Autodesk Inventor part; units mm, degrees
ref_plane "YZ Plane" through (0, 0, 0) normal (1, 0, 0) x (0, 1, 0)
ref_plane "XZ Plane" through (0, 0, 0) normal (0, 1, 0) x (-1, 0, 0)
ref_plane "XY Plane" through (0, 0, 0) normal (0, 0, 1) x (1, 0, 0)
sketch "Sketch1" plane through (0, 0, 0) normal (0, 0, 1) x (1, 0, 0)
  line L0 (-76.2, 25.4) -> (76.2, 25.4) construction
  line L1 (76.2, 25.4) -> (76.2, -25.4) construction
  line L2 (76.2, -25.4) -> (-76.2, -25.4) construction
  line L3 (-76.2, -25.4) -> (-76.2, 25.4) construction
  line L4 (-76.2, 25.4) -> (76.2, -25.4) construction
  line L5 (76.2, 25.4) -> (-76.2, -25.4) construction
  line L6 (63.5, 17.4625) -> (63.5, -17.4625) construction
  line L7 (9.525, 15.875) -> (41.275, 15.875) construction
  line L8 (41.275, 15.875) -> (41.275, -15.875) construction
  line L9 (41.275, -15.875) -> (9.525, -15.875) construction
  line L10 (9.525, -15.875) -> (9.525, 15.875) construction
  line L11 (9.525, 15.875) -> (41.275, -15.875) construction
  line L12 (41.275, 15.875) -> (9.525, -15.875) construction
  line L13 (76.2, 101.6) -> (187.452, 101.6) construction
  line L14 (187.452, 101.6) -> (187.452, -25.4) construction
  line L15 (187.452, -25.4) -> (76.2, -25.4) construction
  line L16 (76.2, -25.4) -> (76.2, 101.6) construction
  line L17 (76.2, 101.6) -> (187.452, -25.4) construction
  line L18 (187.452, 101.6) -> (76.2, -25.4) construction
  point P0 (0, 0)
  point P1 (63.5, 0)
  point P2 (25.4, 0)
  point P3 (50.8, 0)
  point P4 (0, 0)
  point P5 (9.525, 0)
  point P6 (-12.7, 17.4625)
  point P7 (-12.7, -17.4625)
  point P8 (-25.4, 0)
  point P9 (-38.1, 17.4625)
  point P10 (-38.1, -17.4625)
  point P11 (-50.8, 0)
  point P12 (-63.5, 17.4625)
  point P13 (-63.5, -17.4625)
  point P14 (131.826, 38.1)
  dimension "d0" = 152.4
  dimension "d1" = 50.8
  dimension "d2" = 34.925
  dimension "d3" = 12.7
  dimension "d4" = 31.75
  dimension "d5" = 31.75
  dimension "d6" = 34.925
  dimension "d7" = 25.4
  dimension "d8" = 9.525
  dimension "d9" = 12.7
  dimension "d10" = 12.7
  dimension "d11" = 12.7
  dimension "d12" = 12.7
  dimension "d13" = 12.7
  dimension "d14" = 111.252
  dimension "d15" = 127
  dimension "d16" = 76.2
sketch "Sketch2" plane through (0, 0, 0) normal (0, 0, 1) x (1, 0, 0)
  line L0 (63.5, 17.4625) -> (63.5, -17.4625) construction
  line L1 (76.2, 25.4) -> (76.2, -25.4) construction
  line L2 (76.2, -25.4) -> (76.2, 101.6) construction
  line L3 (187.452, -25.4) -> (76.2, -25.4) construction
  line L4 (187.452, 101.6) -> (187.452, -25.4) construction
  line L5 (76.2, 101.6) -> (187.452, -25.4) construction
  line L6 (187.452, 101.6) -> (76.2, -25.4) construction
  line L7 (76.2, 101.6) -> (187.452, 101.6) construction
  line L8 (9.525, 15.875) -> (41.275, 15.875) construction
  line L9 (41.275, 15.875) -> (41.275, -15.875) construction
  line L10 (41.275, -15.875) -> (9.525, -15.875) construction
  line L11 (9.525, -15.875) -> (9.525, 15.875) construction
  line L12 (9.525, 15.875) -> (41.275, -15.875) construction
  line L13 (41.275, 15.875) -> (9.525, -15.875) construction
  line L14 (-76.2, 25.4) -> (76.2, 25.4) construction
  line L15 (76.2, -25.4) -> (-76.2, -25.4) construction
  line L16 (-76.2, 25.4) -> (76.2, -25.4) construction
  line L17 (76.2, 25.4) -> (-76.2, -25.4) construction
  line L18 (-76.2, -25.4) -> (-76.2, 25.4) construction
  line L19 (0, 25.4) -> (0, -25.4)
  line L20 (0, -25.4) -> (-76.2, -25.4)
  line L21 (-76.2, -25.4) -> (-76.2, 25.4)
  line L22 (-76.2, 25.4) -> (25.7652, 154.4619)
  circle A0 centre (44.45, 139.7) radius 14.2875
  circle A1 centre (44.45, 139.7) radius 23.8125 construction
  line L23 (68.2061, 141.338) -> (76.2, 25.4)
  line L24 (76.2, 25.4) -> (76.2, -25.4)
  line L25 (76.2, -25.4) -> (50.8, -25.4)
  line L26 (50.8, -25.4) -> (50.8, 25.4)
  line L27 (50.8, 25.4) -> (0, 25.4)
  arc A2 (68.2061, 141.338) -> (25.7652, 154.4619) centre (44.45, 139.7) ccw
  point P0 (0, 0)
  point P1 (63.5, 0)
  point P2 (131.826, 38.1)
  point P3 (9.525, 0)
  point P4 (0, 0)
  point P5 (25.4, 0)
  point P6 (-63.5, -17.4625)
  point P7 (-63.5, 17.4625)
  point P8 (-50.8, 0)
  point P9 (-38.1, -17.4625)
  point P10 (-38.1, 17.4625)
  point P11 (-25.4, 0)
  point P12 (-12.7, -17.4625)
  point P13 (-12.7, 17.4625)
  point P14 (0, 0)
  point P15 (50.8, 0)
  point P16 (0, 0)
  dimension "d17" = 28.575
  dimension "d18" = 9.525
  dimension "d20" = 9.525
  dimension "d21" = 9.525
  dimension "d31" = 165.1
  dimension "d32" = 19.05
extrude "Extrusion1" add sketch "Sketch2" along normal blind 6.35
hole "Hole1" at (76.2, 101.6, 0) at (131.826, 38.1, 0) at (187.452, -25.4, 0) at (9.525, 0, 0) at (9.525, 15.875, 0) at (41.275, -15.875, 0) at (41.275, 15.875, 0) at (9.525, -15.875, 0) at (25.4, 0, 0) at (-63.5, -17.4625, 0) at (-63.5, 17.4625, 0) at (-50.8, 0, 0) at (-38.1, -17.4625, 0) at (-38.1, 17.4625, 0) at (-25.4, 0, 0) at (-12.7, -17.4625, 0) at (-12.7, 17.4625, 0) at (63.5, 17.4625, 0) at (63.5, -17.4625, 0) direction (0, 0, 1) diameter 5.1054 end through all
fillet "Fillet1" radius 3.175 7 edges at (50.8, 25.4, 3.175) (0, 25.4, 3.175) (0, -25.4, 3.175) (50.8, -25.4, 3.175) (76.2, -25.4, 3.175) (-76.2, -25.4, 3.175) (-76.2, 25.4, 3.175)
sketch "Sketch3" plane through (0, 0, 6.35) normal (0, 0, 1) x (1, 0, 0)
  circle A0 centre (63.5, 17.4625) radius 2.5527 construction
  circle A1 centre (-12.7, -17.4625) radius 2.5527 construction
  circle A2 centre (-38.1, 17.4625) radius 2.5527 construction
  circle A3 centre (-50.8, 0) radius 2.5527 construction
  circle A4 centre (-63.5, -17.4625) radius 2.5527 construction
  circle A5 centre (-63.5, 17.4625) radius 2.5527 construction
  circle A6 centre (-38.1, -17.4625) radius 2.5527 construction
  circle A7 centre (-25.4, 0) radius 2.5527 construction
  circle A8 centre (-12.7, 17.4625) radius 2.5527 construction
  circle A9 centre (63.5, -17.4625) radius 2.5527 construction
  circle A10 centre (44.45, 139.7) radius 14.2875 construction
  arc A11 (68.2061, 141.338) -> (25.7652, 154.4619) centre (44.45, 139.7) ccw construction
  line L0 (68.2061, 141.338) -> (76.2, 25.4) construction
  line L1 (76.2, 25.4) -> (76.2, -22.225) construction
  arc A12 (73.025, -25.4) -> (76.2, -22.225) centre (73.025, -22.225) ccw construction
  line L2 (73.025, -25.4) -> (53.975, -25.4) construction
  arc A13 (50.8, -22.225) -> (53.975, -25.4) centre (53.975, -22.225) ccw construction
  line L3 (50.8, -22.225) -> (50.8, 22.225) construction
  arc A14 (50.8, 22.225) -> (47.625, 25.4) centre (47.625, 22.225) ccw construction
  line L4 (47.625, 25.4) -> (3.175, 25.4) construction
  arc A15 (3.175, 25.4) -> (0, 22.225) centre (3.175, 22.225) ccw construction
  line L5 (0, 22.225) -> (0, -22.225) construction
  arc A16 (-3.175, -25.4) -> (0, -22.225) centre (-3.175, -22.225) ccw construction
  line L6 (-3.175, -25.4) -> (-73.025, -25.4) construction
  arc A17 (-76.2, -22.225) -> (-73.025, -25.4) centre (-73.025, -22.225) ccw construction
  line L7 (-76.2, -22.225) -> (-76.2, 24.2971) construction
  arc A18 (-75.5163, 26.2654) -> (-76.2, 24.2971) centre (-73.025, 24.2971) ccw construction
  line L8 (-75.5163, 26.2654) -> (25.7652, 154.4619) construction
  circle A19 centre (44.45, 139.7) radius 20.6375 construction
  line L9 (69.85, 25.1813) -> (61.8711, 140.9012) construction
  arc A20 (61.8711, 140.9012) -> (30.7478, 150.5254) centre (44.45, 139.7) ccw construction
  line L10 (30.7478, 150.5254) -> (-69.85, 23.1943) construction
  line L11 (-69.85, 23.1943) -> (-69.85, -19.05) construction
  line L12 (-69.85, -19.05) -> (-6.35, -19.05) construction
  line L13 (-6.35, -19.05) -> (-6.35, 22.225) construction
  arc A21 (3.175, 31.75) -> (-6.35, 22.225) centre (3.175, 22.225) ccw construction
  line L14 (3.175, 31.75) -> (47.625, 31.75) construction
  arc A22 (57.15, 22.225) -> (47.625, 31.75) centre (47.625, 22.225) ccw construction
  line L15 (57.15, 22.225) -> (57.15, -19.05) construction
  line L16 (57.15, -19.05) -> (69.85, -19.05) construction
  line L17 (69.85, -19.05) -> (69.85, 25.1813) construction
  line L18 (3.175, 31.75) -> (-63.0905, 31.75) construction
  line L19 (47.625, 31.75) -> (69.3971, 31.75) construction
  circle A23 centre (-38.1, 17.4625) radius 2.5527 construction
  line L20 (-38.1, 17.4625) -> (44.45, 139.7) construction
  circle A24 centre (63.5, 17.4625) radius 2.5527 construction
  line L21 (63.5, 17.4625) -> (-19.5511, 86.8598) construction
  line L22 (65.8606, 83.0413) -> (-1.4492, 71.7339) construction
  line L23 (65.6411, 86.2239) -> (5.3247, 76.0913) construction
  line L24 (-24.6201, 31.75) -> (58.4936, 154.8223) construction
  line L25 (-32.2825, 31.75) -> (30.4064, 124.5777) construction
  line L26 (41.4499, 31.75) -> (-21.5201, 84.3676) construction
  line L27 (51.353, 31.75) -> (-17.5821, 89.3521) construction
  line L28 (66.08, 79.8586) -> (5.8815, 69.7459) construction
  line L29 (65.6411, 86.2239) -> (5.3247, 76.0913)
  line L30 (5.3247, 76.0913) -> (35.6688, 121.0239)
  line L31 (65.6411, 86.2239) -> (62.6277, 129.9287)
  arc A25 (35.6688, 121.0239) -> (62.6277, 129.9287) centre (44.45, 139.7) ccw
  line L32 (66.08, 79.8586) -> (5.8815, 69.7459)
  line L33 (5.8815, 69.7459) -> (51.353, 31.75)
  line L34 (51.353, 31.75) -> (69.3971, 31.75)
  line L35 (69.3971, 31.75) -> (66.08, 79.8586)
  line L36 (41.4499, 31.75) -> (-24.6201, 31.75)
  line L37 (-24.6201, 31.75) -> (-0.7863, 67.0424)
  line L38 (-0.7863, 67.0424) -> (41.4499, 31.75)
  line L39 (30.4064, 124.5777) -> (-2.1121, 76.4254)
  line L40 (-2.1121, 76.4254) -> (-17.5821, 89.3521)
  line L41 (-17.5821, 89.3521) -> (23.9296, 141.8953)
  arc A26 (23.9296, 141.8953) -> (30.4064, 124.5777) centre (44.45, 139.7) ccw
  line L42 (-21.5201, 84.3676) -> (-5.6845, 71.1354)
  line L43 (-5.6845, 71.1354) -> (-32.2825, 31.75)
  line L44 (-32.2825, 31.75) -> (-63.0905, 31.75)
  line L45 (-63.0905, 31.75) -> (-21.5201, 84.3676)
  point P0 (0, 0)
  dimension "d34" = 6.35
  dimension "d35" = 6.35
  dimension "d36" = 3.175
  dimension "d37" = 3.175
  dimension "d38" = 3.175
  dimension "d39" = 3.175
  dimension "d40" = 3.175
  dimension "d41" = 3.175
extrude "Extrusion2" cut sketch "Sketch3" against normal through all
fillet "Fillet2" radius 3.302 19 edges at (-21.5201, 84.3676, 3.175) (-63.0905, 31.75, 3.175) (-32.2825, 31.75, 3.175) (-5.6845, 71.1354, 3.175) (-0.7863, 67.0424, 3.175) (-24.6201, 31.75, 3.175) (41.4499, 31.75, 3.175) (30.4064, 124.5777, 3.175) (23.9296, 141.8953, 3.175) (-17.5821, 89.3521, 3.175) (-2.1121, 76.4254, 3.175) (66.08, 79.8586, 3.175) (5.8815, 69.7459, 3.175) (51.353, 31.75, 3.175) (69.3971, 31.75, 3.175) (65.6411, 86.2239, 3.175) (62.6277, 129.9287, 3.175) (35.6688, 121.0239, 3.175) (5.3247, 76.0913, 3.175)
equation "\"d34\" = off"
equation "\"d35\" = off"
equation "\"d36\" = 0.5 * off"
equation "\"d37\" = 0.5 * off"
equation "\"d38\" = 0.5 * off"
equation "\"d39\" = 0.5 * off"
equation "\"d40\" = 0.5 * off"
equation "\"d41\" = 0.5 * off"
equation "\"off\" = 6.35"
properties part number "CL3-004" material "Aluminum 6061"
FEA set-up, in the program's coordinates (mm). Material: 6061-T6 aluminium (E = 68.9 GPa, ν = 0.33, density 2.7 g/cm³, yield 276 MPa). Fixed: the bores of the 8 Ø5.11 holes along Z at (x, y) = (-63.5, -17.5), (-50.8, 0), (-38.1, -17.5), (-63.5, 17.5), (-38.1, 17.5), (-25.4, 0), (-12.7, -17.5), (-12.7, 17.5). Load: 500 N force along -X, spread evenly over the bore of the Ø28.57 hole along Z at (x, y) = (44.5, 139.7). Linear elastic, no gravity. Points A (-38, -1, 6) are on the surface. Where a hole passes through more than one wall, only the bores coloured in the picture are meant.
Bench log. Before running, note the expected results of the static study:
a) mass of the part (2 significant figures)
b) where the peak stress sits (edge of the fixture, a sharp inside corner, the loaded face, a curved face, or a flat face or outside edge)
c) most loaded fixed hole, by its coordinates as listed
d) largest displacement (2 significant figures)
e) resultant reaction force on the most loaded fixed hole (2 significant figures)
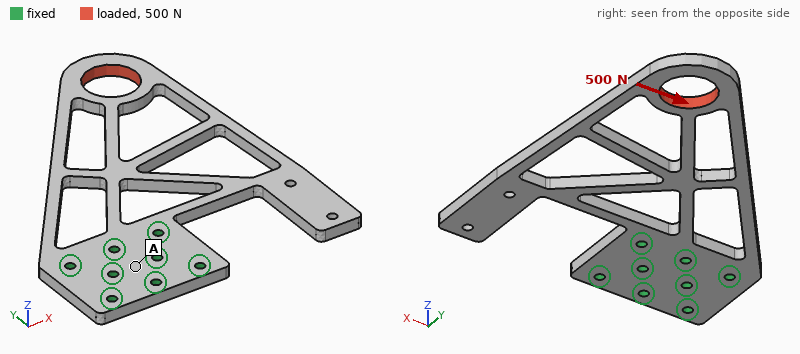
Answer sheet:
170 g
a curved face
(-63.5, 17.5)
0.69 mm
1.2 kN
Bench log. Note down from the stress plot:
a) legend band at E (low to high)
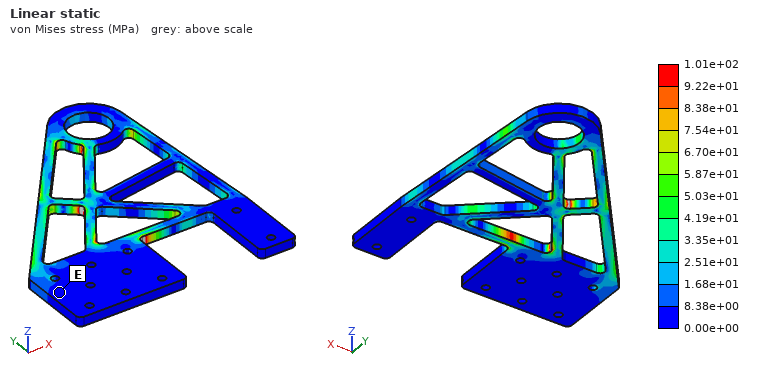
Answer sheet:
0.00e+00 to 8.38e+00 MPa
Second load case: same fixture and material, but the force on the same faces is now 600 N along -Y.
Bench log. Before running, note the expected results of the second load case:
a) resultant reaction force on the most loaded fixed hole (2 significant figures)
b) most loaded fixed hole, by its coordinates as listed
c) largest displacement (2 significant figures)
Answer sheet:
810 N
(-63.5, 17.5)
0.66 mm
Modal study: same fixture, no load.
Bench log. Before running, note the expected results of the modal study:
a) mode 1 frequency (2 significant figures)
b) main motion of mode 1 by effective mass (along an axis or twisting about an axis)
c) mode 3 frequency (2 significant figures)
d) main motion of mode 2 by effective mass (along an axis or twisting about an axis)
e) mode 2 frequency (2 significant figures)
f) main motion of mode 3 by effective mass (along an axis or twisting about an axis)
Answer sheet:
160 Hz
along Z
560 Hz
along Z
290 Hz
along Y
